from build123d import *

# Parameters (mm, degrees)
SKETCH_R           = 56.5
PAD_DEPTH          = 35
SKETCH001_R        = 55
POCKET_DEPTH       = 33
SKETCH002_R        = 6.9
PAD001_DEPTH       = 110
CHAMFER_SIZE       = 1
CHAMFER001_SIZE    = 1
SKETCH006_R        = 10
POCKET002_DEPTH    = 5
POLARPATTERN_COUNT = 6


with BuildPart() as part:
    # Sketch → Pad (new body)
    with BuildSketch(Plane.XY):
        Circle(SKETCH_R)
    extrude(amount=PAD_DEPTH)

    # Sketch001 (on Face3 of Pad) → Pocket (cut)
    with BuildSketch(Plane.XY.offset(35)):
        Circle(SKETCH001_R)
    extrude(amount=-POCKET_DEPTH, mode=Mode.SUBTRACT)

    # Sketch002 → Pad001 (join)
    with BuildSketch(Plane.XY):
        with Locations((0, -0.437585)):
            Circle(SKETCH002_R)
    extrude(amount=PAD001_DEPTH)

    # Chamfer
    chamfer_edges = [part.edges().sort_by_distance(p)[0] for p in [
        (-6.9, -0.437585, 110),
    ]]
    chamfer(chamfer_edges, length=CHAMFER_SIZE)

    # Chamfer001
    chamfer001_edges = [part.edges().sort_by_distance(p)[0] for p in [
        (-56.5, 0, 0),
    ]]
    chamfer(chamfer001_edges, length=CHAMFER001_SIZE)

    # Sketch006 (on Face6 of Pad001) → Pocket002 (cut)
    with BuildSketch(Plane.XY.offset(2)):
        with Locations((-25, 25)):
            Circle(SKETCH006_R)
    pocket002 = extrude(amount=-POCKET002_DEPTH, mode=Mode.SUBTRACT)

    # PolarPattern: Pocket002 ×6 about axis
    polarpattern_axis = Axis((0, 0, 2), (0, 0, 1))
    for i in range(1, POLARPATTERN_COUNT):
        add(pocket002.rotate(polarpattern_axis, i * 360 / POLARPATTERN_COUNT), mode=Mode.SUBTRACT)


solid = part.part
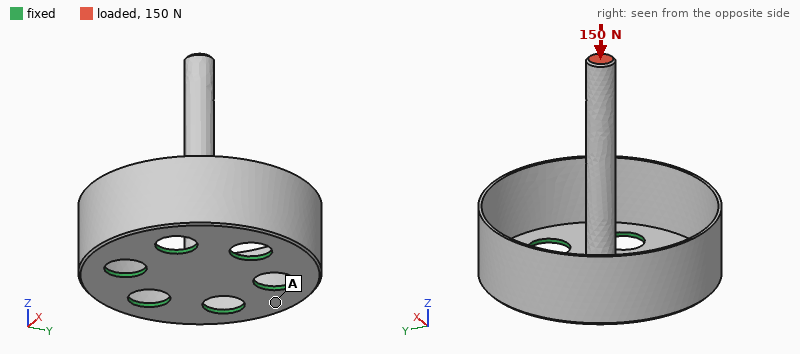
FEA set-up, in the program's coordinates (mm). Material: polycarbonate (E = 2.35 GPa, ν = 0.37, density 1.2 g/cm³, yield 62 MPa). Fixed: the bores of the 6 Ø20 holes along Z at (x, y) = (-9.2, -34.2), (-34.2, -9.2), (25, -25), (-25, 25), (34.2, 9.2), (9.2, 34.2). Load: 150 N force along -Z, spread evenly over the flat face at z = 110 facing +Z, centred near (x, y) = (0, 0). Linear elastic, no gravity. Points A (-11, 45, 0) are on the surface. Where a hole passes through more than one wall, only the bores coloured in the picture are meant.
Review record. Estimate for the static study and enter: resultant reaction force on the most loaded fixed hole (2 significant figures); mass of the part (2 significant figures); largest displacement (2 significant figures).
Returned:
29 N
60 g
0.63 mm
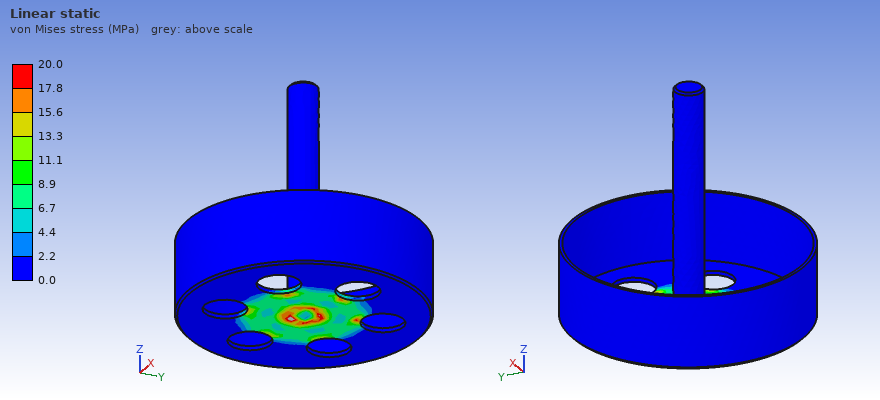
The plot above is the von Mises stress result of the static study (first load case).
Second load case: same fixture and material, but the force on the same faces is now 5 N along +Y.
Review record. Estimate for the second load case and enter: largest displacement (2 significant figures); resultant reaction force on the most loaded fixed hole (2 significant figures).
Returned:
2.0 mm
9.4 N
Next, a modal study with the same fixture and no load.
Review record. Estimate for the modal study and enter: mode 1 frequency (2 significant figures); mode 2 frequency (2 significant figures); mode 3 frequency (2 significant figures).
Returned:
100 Hz
100 Hz
450 Hz
